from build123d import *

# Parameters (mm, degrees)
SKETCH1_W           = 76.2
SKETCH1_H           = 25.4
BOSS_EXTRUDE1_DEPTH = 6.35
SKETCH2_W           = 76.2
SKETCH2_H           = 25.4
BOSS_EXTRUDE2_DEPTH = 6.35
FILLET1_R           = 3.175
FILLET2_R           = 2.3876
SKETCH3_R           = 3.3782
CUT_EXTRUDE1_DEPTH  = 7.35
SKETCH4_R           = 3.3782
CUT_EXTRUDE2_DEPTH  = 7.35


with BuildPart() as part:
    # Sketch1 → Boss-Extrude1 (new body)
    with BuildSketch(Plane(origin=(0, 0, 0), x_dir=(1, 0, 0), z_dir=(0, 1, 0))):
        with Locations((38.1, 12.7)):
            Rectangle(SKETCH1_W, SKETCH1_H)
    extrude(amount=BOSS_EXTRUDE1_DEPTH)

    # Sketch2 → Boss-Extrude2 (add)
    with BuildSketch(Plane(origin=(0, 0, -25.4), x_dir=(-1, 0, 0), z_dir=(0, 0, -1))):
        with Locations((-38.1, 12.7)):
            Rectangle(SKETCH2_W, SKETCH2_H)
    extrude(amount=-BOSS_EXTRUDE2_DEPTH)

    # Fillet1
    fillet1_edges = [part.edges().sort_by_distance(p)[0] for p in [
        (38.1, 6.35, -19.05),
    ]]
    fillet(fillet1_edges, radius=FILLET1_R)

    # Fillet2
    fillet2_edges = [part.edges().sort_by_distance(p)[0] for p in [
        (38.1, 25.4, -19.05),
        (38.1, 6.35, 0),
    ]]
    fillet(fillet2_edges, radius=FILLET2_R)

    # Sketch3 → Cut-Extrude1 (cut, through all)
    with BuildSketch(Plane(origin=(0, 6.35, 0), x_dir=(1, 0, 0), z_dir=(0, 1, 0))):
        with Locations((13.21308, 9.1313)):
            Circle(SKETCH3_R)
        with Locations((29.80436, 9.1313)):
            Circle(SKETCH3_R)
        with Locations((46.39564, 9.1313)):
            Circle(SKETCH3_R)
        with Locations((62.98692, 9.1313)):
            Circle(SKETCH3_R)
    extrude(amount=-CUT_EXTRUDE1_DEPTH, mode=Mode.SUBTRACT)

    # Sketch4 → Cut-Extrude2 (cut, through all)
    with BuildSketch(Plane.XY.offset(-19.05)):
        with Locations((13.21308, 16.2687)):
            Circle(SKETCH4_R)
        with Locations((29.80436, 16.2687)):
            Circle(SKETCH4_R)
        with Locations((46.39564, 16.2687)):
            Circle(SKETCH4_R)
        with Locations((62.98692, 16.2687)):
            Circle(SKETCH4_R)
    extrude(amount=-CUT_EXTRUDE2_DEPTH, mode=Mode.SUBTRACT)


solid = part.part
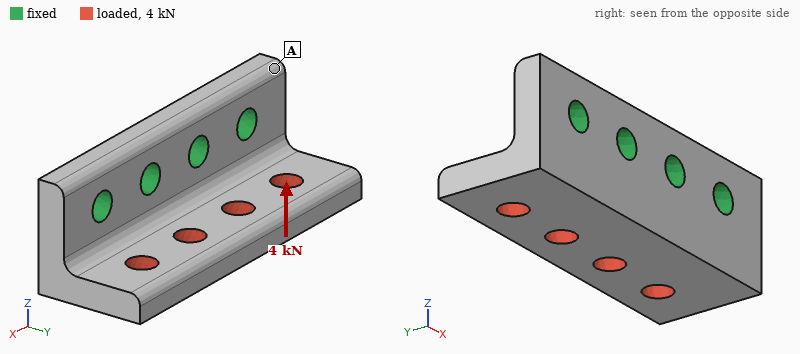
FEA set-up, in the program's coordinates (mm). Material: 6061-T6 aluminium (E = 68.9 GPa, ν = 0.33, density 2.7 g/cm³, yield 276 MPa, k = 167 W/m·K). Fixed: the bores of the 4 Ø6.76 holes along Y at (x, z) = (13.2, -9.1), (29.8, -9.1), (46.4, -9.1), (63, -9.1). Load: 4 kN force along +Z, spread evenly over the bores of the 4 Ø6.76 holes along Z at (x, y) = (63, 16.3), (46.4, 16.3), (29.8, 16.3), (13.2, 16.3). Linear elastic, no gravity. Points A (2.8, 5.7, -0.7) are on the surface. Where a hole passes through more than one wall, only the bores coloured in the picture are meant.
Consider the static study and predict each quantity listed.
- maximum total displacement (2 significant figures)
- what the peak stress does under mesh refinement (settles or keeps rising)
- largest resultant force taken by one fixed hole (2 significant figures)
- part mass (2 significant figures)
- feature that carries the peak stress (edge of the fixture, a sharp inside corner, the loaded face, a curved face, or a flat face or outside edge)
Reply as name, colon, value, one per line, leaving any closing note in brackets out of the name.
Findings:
maximum total displacement: 0.14 mm
what the peak stress does under mesh refinement: keeps rising
largest resultant force taken by one fixed hole: 1.0 kN
part mass: 53 g
feature that carries the peak stress: edge of the fixture
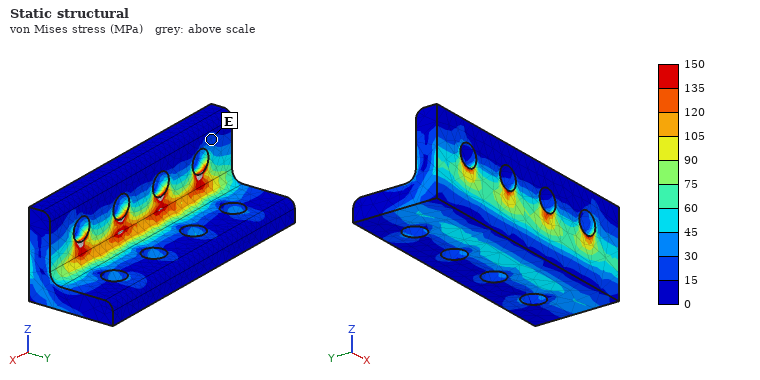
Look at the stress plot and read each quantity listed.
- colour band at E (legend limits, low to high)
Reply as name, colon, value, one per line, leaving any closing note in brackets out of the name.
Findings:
colour band at E: 15 to 30 MPa
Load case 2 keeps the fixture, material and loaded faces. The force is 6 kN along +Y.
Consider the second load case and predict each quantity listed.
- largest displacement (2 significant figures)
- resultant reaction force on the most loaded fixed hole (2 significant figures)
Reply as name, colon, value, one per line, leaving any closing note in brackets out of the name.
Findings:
largest displacement: 93 µm
resultant reaction force on the most loaded fixed hole: 1.5 kN
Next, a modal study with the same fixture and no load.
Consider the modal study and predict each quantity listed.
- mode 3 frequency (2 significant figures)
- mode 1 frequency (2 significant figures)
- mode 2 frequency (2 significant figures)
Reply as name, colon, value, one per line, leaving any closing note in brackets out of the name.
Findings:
mode 3 frequency: 14 kHz
mode 1 frequency: 6500 Hz
mode 2 frequency: 8000 Hz
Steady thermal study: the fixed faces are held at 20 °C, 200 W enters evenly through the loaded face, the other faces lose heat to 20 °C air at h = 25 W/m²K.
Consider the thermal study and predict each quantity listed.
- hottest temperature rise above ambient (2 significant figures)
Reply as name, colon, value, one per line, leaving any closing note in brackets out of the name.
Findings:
hottest temperature rise above ambient: 65 K
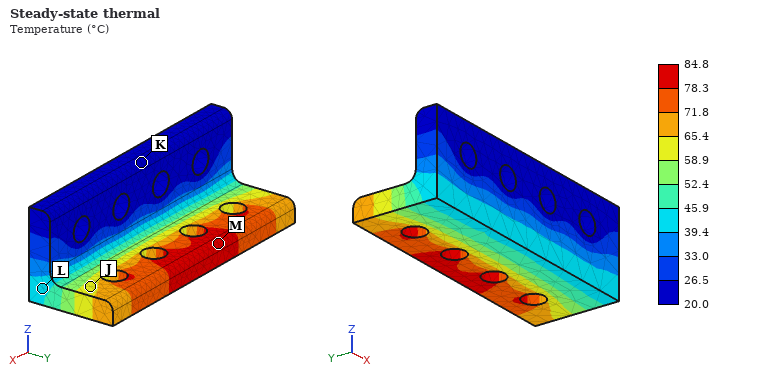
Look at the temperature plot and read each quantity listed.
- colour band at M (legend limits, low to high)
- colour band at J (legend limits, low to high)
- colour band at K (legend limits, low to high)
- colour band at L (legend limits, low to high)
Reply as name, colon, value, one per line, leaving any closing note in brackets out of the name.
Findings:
colour band at M: 78.3 to 84.8 °C
colour band at J: 58.9 to 65.4 °C
colour band at K: 20.0 to 26.5 °C
colour band at L: 39.4 to 45.9 °C
